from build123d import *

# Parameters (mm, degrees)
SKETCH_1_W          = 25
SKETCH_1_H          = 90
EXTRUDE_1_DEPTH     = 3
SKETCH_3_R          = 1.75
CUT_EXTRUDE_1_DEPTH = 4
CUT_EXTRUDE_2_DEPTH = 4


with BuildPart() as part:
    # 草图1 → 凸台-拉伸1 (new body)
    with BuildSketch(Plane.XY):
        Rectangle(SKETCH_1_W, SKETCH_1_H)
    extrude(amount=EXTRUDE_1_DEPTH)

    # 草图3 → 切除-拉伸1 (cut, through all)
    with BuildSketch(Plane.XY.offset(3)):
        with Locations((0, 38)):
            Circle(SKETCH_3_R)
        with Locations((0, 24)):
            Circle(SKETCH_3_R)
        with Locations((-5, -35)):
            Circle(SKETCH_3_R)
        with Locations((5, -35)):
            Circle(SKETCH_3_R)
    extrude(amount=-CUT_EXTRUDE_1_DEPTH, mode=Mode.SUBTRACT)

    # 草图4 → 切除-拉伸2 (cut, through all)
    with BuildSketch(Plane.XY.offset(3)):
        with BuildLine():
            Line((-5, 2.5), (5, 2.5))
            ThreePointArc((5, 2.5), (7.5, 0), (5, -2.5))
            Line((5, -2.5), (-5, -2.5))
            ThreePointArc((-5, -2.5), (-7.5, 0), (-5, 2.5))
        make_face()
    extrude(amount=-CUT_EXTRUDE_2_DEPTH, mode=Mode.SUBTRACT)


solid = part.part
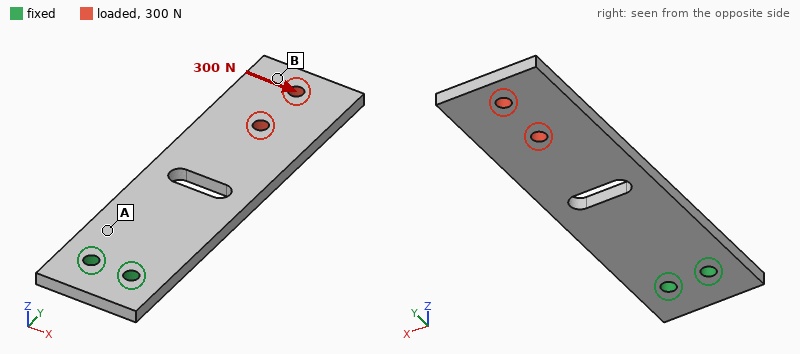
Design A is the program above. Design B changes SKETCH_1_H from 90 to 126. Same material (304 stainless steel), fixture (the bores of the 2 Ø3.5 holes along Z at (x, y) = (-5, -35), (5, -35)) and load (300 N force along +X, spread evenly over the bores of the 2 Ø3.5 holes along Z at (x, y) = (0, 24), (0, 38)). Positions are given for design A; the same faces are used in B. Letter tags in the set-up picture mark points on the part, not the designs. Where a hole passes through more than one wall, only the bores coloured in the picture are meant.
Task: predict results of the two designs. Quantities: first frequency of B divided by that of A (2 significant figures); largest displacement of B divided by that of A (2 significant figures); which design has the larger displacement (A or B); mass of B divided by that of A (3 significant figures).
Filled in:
0.65
1.3
B
1.42
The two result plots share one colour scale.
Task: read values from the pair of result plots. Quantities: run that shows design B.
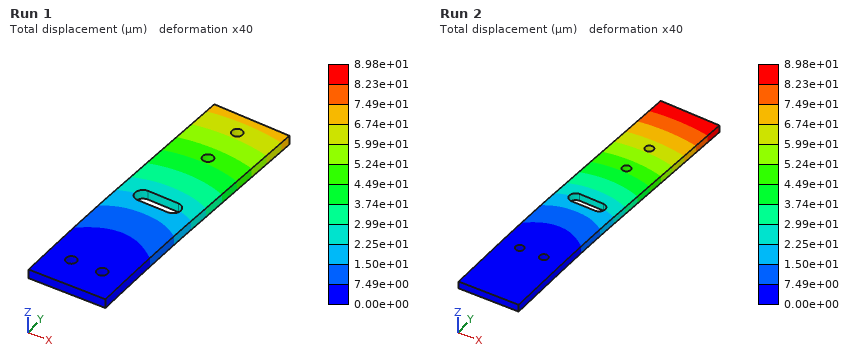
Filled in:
Run 2
